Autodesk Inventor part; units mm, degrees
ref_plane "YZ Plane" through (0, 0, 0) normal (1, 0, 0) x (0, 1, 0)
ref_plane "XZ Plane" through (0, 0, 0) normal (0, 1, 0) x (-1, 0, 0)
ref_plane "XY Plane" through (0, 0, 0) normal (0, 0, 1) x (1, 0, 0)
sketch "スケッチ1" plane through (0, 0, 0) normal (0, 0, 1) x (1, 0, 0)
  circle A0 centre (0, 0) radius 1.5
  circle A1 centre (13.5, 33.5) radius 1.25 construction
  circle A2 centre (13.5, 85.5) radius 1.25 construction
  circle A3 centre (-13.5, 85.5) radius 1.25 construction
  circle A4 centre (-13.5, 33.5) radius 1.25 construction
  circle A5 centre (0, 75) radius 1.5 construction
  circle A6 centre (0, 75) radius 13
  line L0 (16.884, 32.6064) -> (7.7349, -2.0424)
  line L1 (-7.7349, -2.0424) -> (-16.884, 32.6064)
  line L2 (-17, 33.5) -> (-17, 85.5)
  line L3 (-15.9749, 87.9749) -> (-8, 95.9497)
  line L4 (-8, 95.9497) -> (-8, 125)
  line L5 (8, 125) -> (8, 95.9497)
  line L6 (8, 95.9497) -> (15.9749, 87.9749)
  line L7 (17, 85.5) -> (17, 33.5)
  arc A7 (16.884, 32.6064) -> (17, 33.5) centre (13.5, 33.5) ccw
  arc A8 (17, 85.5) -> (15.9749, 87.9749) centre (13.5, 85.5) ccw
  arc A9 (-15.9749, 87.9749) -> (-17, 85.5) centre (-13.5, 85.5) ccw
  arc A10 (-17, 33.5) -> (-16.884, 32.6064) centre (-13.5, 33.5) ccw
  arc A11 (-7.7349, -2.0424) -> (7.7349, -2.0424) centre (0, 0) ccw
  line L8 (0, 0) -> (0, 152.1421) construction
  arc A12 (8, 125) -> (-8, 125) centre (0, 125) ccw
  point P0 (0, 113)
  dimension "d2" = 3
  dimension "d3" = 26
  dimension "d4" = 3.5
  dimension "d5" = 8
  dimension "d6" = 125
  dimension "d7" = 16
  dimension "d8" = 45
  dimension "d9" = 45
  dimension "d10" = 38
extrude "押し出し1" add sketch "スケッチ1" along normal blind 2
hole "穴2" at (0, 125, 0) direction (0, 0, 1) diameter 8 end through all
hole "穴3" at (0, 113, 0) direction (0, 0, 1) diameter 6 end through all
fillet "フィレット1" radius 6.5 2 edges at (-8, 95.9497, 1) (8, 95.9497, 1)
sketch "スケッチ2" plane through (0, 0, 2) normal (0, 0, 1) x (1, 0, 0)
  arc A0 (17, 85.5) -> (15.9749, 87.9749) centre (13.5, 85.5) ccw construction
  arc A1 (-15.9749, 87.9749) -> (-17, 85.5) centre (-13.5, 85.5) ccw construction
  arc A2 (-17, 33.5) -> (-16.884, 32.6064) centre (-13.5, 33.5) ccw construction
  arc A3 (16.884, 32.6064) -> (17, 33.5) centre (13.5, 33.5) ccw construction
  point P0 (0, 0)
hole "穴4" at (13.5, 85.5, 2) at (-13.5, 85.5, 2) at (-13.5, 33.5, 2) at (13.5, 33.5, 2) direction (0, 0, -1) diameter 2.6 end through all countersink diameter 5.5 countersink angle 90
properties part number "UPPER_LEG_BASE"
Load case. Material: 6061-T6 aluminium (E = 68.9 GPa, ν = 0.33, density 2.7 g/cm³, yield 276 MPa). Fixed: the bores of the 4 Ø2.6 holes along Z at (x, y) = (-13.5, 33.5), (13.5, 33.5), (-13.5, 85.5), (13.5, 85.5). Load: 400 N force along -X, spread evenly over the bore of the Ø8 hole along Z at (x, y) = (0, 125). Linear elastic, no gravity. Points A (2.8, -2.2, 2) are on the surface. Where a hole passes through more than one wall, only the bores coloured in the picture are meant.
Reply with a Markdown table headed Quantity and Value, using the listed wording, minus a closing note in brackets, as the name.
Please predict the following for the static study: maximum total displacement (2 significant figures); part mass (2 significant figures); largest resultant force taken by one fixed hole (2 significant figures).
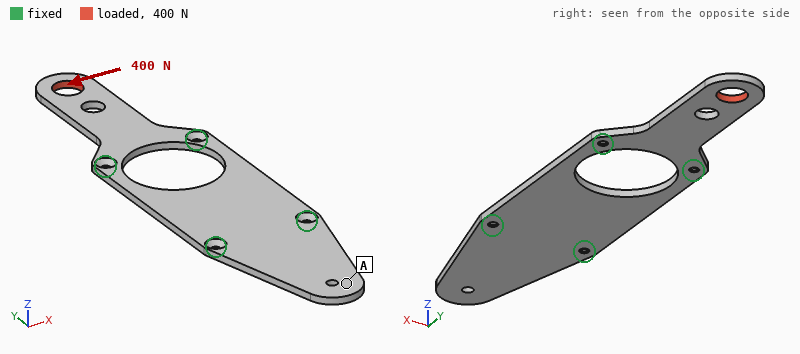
| Quantity | Value |
|---|---|
| maximum total displacement | 0.23 mm |
| part mass | 16 g |
| largest resultant force taken by one fixed hole | 630 N |
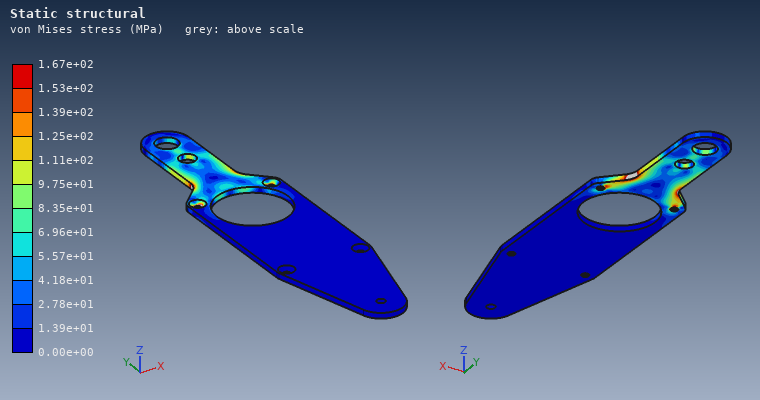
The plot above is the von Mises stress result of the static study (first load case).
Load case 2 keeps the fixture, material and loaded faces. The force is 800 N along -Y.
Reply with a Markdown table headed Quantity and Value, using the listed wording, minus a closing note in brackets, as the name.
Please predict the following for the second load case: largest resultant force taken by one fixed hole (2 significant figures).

| Quantity | Value |
|---|---|
| largest resultant force taken by one fixed hole | 450 N |
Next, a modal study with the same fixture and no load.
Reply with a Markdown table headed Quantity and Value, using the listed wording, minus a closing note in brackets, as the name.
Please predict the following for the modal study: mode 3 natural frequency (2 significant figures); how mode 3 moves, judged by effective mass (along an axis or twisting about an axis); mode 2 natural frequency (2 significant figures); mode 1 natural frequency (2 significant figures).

| Quantity | Value |
|---|---|
| mode 3 natural frequency | 2800 Hz |
| how mode 3 moves, judged by effective mass | along Z |
| mode 2 natural frequency | 1100 Hz |
| mode 1 natural frequency | 720 Hz |
